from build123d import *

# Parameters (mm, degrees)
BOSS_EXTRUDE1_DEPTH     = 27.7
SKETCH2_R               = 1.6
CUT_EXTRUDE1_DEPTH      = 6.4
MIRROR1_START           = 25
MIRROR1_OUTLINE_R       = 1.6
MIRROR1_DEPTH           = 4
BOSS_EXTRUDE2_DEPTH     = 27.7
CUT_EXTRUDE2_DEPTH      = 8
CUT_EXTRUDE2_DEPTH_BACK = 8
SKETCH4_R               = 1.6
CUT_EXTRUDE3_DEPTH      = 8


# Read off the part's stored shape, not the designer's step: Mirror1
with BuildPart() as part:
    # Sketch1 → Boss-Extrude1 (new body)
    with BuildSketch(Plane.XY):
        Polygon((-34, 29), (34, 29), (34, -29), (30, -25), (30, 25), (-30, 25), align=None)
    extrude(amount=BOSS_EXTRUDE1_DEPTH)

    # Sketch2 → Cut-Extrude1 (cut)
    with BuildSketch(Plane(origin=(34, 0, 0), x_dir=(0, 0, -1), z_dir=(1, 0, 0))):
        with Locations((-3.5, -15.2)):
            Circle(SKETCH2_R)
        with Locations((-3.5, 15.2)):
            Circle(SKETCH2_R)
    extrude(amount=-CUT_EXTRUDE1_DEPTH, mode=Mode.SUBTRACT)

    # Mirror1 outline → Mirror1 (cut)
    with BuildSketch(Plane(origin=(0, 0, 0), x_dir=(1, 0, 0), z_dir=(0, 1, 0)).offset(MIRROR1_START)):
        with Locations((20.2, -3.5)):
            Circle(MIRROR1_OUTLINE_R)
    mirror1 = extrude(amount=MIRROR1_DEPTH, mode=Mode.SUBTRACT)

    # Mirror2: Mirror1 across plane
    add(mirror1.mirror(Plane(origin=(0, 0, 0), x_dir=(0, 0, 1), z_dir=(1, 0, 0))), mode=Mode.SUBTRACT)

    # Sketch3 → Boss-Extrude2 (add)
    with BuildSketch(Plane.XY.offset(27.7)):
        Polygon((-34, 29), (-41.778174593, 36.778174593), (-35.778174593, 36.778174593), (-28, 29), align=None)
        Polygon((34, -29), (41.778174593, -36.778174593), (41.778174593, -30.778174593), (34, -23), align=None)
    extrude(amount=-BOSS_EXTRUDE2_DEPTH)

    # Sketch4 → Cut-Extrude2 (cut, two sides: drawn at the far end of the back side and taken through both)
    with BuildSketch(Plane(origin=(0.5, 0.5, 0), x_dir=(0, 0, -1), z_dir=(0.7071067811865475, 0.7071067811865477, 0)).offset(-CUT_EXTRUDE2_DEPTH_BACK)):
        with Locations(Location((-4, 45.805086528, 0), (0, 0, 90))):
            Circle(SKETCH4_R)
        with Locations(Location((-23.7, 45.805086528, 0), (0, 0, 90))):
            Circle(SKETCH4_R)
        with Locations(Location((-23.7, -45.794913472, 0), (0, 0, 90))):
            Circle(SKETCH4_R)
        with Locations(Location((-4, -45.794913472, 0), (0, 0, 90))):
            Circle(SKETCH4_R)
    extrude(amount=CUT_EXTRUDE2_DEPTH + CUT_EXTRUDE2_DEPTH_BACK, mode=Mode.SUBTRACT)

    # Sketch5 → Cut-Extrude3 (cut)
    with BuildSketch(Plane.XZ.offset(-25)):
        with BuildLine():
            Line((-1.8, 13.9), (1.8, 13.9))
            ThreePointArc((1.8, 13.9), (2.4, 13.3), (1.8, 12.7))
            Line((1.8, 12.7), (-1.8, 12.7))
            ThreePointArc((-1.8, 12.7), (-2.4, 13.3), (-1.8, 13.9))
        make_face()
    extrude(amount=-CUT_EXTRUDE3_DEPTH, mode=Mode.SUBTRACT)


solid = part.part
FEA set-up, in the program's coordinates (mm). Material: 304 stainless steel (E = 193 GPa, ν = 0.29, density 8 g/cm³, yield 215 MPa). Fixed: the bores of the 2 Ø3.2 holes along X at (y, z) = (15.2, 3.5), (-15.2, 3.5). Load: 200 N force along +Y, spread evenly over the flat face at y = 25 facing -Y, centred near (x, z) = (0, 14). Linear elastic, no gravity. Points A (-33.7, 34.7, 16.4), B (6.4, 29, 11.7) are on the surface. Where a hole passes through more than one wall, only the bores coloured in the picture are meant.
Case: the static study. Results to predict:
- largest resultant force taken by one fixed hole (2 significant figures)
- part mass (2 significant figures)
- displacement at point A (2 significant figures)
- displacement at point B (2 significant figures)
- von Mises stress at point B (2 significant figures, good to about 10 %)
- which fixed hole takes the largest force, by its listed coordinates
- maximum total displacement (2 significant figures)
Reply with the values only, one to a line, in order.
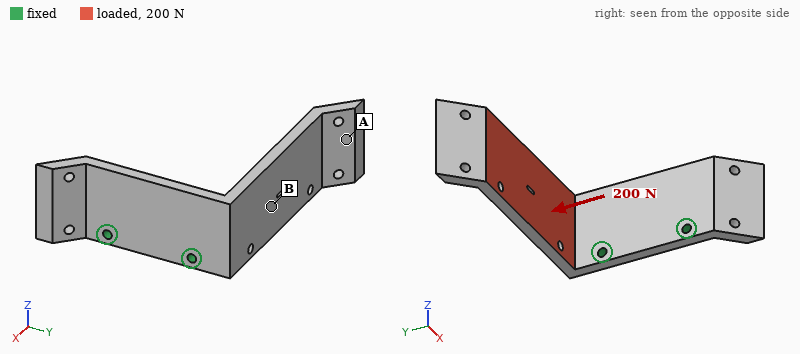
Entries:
180 N
120 g
0.44 mm
0.14 mm
28 MPa
(15.2, 3.5)
0.50 mm
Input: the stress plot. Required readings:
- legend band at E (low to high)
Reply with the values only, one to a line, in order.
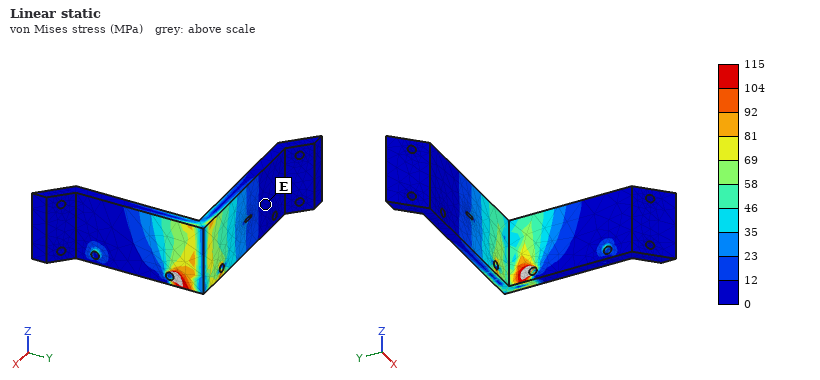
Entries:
0 to 12 MPa
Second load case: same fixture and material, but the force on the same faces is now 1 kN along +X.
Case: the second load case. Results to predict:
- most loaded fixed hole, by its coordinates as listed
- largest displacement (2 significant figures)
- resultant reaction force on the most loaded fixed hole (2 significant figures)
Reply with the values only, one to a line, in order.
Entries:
(15.2, 3.5)
0.27 mm
1.1 kN
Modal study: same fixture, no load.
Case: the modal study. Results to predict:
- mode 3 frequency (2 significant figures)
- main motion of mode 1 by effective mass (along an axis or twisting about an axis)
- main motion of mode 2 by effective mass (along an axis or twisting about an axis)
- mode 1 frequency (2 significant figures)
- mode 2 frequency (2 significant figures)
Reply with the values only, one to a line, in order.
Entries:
2800 Hz
along Y
along Z
430 Hz
720 Hz
